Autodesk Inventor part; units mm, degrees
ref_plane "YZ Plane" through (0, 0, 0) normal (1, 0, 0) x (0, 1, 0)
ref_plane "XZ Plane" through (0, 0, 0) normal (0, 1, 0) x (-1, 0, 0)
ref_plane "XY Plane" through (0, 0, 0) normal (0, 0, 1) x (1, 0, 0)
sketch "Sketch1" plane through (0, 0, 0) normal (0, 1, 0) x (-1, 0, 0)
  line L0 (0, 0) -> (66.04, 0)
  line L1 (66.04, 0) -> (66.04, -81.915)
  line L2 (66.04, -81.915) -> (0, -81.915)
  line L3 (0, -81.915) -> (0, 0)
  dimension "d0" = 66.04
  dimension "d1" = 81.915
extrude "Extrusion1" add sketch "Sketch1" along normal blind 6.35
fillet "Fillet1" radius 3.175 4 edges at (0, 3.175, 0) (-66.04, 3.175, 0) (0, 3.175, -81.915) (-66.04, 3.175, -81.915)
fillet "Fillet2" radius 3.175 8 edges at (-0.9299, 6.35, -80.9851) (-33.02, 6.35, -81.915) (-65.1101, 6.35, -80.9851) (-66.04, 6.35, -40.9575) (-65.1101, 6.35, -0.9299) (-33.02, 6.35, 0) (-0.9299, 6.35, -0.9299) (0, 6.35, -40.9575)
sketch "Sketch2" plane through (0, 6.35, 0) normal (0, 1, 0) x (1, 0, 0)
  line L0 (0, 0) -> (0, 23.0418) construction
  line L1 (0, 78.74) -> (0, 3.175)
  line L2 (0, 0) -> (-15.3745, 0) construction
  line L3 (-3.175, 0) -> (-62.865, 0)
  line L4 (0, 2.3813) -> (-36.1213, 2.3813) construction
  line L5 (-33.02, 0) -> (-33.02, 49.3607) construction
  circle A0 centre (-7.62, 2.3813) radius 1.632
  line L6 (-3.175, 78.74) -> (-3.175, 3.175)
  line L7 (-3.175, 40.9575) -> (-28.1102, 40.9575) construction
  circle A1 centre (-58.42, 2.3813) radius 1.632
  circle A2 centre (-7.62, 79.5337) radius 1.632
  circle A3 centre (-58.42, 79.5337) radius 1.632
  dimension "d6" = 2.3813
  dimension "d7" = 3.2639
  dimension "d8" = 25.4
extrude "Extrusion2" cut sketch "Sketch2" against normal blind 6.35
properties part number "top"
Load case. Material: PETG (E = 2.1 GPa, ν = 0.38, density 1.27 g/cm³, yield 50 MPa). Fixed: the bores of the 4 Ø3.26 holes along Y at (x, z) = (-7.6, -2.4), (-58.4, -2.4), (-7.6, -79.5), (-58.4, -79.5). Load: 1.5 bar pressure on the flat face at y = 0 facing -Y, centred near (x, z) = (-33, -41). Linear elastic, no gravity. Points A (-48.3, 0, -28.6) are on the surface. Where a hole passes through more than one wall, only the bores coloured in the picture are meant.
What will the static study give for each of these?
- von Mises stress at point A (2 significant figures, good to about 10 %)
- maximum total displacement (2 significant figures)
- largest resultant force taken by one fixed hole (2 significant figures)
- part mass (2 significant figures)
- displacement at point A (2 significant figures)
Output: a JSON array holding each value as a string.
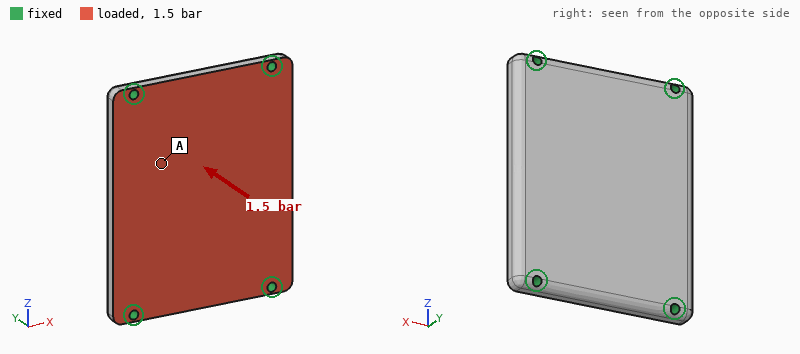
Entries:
["5.4 MPa", "0.58 mm", "200 N", "43 g", "0.48 mm"]
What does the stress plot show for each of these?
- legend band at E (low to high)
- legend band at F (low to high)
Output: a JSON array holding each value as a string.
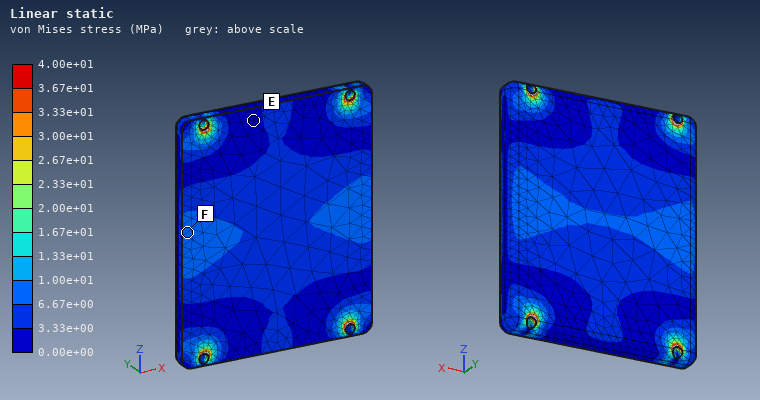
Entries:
["0.00e+00 to 3.33e+00 MPa", "6.67e+00 to 1.00e+01 MPa"]
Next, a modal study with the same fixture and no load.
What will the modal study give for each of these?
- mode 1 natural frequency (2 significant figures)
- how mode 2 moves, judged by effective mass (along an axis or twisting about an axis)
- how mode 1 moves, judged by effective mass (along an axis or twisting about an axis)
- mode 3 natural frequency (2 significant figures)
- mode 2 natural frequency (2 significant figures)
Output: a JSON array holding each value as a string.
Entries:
["1000 Hz", "twisting about Z", "along Y", "2500 Hz", "1600 Hz"]
